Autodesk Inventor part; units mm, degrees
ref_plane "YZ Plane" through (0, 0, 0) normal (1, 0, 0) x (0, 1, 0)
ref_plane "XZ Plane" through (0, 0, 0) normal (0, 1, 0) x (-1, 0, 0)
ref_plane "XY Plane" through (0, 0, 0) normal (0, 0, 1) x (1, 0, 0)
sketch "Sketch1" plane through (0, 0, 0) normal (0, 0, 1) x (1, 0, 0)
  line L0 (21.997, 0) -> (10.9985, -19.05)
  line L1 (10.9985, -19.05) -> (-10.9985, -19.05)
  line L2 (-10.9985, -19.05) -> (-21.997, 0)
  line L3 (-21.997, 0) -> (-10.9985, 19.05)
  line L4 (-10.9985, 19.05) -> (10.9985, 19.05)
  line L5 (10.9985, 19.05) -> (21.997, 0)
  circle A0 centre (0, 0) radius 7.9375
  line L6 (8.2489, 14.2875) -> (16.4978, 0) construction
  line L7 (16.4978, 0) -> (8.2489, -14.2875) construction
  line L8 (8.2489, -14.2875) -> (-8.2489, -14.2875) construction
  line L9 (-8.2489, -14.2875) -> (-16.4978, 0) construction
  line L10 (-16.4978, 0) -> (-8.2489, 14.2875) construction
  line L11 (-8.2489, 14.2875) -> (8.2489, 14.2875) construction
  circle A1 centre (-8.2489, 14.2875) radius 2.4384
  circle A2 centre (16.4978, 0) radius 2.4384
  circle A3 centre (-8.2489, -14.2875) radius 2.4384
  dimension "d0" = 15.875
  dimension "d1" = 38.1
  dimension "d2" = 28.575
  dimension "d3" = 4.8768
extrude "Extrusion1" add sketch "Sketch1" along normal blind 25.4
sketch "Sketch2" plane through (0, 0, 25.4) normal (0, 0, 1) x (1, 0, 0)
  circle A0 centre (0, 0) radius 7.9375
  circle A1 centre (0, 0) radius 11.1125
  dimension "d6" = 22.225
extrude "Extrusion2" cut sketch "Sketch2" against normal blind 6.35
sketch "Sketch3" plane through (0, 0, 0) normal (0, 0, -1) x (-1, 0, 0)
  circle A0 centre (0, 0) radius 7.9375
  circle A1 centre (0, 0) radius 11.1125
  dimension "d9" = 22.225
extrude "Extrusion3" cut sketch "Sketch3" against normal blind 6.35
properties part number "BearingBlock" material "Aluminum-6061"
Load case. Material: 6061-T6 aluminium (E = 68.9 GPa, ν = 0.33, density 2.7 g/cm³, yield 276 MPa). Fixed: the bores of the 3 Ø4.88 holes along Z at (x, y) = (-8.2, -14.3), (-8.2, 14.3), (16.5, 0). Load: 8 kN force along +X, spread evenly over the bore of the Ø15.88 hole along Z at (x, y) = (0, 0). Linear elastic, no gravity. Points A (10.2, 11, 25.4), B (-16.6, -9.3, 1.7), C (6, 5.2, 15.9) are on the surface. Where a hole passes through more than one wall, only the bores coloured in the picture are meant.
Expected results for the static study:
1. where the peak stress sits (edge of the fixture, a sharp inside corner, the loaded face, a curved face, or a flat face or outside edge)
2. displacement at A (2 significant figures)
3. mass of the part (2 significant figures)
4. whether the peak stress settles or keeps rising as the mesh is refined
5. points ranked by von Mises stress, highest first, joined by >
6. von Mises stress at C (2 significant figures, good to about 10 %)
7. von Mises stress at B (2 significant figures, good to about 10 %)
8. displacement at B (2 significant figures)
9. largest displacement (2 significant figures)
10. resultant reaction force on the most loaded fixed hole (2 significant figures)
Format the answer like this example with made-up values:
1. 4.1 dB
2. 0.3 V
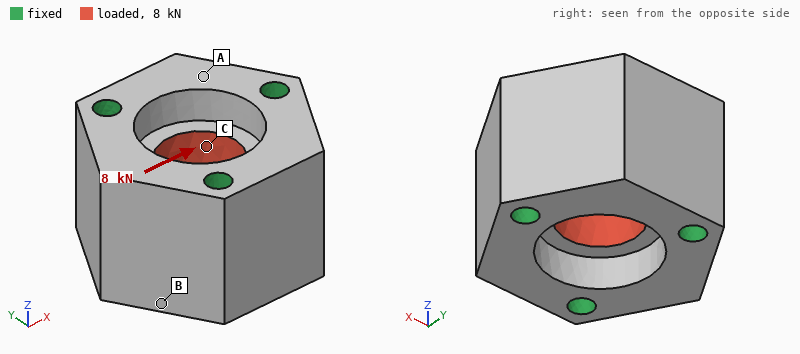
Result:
1. edge of the fixture
2. 0.99 µm
3. 62 g
4. keeps rising
5. C > B > A
6. 16 MPa
7. 6.8 MPa
8. 1.1 µm
9. 3.7 µm
10. 2.9 kN
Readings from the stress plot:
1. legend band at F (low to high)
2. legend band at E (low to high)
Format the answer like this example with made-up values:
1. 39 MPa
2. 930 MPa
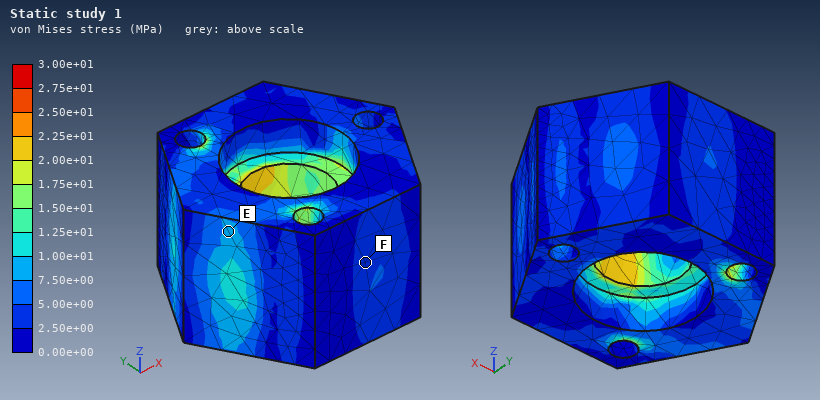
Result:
1. 2.50e+00 to 5.00e+00 MPa
2. 7.50e+00 to 1.00e+01 MPa
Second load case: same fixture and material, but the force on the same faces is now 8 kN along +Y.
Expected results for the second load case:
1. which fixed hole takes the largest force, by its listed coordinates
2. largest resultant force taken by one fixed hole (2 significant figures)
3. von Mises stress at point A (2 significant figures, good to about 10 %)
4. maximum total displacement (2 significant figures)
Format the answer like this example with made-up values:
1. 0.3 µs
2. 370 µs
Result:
1. (16.5, 0)
2. 3.0 kN
3. 3.3 MPa
4. 3.4 µm
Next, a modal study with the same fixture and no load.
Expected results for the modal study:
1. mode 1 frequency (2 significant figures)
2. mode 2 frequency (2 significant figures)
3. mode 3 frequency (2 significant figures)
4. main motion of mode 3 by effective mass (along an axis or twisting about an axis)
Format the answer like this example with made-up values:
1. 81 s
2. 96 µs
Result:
1. 39 kHz
2. 39 kHz
3. 42 kHz
4. along Z
